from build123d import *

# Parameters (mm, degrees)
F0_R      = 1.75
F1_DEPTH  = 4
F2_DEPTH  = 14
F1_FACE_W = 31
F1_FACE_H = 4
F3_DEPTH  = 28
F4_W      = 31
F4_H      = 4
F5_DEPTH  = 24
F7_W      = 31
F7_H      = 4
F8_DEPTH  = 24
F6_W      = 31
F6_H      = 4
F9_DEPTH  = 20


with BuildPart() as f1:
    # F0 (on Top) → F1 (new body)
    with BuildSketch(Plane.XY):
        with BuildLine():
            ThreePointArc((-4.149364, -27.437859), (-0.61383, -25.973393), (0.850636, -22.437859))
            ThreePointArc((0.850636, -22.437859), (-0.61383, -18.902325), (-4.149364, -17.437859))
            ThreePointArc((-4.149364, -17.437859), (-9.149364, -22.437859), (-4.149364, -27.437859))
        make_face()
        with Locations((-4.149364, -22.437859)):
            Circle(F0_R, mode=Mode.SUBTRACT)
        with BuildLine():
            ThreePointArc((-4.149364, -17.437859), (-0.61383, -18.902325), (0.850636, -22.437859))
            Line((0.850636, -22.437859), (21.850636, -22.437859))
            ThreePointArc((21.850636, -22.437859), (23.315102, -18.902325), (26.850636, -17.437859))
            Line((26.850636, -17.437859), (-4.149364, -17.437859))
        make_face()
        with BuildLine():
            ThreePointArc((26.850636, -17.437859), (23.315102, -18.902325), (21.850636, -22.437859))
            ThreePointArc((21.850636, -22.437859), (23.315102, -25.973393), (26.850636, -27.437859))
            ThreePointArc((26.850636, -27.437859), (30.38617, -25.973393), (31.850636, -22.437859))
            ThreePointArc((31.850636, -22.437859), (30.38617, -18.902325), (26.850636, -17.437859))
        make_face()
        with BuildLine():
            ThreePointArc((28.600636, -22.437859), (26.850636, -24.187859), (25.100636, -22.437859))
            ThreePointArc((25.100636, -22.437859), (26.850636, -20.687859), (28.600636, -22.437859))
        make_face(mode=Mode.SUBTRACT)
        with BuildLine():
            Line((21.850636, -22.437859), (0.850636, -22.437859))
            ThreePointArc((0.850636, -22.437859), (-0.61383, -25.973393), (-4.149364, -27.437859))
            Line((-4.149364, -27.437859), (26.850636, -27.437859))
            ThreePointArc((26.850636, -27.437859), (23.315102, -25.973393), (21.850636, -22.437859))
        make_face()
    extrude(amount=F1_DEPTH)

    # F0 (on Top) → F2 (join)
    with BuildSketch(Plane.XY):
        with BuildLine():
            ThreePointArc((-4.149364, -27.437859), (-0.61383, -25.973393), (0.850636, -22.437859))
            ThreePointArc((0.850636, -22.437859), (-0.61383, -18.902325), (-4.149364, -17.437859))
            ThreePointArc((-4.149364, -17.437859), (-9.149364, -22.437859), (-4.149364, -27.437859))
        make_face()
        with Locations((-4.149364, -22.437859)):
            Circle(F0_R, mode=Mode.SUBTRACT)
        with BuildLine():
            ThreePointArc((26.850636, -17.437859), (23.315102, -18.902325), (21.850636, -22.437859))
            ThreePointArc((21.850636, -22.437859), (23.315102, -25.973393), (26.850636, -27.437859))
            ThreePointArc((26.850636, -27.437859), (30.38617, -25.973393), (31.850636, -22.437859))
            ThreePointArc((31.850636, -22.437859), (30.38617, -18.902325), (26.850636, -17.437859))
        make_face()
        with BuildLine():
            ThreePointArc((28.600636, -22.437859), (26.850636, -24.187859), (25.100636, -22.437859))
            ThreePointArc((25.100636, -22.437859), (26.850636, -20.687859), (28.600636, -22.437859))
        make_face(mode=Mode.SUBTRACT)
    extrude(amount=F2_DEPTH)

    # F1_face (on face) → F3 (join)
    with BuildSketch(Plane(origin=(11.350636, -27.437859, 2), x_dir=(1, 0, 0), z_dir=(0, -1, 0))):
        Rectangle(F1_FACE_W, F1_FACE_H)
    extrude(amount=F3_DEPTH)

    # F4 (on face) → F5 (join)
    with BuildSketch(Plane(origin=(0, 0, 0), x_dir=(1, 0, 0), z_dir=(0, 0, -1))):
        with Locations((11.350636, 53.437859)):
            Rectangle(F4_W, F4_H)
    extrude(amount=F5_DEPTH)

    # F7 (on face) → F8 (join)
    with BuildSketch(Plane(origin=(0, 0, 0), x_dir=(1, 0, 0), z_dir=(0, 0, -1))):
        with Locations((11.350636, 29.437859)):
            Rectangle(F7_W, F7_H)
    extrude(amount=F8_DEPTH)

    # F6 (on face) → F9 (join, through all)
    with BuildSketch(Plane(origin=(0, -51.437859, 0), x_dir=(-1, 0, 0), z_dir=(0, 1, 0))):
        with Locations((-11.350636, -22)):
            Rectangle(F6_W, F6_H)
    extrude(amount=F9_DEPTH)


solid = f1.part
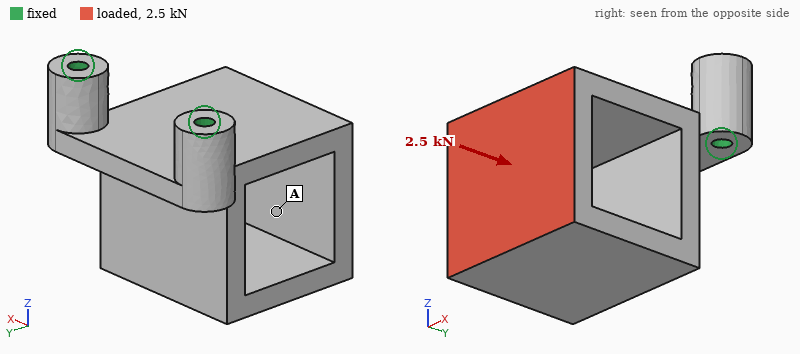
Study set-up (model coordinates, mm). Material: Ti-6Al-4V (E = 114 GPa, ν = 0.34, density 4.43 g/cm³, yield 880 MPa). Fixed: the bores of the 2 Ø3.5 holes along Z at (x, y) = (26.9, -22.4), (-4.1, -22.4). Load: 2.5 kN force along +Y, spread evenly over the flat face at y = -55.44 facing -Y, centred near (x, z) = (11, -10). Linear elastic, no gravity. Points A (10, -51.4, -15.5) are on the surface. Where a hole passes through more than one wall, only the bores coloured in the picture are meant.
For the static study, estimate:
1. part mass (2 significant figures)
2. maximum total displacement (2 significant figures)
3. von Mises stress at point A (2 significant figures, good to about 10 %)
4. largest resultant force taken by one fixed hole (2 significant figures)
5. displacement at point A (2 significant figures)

65 g
0.53 mm
53 MPa
1.4 kN
0.42 mm
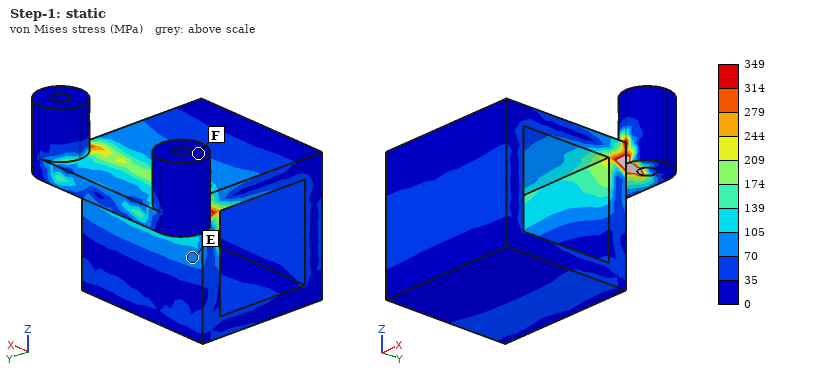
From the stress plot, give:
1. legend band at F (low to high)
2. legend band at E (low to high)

0 to 35 MPa
70 to 105 MPa
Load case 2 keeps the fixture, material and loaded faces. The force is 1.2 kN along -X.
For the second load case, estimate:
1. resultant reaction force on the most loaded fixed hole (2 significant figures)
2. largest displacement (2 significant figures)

1.5 kN
66 µm
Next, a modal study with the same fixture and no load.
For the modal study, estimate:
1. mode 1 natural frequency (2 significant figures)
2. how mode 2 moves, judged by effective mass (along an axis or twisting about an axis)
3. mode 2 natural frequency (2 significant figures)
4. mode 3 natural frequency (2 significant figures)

1400 Hz
along X
4800 Hz
6400 Hz
